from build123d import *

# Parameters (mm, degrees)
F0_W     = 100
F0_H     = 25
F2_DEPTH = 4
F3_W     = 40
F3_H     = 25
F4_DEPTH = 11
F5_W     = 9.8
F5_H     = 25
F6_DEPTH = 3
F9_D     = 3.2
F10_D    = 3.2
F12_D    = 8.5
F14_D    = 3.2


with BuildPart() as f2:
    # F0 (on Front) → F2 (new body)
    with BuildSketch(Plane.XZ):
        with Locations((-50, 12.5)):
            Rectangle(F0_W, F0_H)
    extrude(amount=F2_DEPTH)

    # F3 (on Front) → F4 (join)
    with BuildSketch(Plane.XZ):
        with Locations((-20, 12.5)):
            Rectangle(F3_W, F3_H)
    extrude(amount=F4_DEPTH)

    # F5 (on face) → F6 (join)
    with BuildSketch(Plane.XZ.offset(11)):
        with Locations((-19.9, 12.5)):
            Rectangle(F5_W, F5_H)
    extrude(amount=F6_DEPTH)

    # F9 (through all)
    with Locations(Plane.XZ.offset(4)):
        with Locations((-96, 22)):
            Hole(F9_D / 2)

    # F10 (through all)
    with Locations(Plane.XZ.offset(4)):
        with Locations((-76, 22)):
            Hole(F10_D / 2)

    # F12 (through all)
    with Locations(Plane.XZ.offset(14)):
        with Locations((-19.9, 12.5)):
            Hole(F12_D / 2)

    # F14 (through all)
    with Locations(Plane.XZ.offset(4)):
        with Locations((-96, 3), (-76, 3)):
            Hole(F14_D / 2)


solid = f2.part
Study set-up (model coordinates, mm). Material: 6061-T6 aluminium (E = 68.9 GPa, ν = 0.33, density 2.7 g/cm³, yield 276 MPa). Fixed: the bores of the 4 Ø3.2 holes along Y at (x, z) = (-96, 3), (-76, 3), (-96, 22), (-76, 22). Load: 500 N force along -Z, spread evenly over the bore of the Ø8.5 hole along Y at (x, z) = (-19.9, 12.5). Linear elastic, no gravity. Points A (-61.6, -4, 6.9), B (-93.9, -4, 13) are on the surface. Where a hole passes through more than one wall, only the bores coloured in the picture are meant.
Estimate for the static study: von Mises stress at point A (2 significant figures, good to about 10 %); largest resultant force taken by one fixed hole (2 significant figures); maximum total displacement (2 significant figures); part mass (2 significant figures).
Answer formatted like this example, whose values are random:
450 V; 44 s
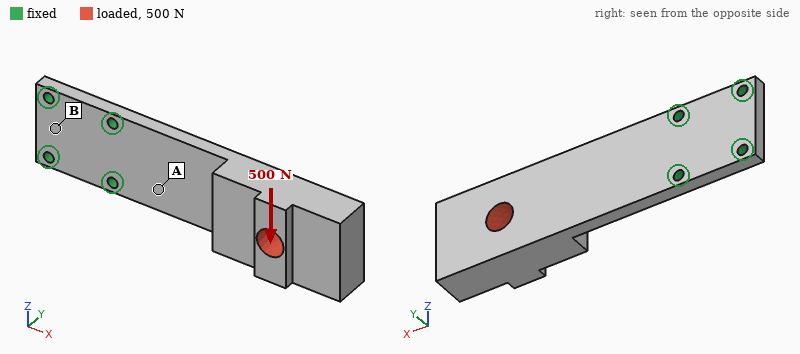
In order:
46 MPa; 1.4 kN; 0.19 mm; 45 g
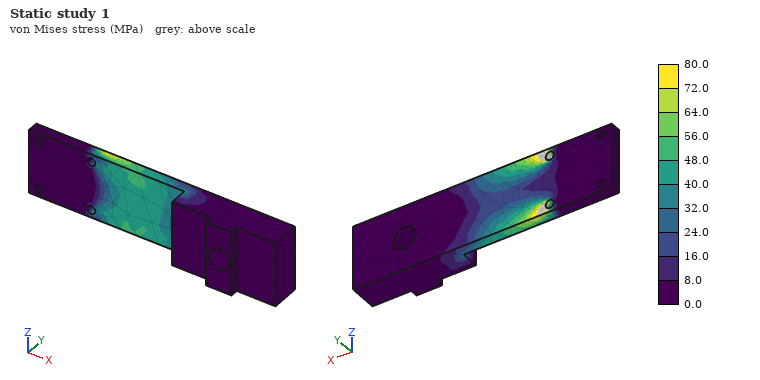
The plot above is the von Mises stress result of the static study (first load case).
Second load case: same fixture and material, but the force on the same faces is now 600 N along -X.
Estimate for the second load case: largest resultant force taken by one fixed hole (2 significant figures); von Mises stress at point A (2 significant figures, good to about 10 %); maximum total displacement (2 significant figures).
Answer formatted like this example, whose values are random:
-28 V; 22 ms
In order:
270 N; 49 MPa; 0.70 mm
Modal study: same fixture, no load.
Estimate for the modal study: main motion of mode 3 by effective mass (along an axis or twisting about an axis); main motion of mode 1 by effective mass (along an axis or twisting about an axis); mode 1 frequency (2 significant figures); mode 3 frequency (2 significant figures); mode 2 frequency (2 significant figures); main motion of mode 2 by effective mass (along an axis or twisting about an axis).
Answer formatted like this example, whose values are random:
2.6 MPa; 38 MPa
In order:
along Z; along Y; 350 Hz; 2600 Hz; 1800 Hz; along Z
